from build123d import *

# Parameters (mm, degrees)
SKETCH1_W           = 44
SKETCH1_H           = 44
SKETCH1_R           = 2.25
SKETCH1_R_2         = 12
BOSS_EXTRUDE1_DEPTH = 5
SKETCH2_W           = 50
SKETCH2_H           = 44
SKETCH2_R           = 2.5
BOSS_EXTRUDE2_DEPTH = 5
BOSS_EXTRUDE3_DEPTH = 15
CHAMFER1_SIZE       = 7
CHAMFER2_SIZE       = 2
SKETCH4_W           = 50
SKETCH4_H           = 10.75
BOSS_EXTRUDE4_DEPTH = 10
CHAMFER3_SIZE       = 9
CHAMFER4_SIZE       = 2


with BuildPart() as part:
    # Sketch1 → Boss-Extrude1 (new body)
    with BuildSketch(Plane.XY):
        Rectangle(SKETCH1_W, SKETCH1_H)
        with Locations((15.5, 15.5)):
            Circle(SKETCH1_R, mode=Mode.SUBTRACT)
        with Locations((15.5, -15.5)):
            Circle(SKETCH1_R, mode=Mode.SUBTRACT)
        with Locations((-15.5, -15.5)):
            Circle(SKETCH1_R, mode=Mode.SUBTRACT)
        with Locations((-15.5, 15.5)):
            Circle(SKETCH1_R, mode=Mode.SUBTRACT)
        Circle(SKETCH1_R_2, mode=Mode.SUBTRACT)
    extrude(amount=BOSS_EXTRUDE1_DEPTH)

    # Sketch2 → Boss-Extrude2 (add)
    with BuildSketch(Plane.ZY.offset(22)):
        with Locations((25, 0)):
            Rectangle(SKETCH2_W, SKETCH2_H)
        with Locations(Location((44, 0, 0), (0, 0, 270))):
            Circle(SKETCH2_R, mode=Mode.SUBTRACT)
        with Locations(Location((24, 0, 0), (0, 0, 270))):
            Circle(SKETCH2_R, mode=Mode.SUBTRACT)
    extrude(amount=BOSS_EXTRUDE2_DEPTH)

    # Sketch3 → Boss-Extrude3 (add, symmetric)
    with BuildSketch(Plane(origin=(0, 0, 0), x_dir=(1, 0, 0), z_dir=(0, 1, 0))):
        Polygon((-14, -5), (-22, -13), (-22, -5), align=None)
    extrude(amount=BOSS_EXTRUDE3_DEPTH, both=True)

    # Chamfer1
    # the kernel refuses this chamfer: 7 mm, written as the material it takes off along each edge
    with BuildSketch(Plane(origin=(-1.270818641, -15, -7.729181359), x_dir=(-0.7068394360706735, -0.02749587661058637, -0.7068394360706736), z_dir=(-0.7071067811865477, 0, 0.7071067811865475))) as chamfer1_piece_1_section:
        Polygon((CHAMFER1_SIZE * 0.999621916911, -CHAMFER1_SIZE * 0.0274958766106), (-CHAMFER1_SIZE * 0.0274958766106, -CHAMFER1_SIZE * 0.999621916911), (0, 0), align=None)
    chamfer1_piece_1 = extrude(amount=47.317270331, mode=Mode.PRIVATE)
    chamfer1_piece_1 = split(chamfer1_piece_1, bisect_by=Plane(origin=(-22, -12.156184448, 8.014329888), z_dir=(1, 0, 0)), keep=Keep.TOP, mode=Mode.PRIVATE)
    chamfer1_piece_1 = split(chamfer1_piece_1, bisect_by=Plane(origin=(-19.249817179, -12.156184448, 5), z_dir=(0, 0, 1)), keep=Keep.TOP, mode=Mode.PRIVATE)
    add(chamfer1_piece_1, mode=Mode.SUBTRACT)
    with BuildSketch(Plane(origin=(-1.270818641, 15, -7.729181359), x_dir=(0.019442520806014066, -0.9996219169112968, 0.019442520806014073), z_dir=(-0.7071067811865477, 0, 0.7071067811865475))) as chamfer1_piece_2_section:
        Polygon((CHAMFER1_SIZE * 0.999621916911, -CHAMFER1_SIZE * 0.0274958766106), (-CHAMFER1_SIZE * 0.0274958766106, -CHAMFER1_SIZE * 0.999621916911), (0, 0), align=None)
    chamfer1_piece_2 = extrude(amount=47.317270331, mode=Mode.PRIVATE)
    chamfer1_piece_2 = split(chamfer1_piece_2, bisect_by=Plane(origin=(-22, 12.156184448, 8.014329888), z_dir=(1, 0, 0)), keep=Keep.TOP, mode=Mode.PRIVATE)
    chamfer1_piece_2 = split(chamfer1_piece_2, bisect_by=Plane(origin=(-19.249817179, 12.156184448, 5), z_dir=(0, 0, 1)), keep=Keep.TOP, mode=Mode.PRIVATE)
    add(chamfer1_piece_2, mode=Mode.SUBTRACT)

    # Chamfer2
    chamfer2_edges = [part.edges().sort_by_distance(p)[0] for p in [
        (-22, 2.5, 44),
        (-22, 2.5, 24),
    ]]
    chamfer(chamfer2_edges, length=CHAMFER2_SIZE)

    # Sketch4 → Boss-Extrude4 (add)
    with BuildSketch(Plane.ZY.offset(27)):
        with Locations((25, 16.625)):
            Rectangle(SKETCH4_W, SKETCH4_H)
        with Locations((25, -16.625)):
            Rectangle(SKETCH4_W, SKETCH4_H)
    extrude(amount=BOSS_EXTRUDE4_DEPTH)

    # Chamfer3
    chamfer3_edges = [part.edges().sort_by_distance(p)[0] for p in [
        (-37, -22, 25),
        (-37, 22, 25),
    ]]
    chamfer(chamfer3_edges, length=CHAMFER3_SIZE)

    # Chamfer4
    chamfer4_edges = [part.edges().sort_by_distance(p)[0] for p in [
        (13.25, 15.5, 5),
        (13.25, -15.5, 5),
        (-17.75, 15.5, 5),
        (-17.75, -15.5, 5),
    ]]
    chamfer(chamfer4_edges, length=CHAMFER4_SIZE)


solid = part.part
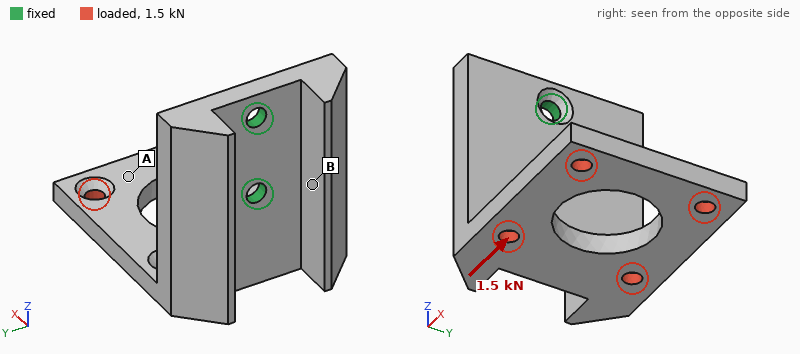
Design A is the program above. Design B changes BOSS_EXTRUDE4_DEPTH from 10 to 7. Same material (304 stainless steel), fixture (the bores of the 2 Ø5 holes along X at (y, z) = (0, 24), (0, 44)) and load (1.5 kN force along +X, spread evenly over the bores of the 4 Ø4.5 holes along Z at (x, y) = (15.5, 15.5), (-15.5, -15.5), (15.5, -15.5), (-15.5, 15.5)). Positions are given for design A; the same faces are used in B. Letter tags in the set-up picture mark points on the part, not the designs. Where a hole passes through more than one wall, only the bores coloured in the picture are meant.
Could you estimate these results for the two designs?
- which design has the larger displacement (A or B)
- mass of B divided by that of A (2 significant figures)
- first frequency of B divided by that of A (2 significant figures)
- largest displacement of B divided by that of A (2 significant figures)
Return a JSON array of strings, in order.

["B", "0.87", "0.95", "1.3"]
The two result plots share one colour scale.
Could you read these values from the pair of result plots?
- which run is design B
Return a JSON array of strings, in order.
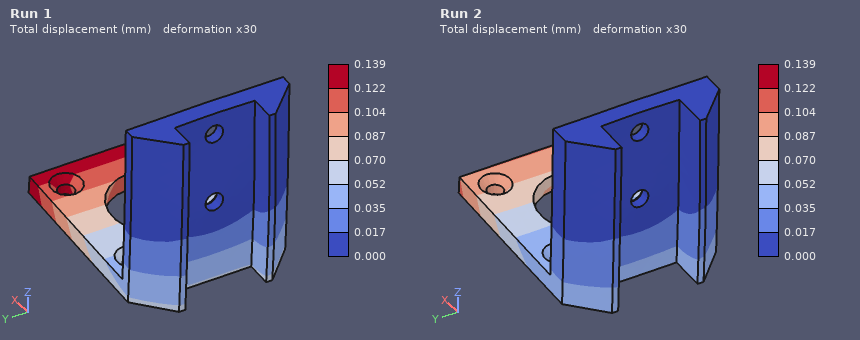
["Run 1"]
